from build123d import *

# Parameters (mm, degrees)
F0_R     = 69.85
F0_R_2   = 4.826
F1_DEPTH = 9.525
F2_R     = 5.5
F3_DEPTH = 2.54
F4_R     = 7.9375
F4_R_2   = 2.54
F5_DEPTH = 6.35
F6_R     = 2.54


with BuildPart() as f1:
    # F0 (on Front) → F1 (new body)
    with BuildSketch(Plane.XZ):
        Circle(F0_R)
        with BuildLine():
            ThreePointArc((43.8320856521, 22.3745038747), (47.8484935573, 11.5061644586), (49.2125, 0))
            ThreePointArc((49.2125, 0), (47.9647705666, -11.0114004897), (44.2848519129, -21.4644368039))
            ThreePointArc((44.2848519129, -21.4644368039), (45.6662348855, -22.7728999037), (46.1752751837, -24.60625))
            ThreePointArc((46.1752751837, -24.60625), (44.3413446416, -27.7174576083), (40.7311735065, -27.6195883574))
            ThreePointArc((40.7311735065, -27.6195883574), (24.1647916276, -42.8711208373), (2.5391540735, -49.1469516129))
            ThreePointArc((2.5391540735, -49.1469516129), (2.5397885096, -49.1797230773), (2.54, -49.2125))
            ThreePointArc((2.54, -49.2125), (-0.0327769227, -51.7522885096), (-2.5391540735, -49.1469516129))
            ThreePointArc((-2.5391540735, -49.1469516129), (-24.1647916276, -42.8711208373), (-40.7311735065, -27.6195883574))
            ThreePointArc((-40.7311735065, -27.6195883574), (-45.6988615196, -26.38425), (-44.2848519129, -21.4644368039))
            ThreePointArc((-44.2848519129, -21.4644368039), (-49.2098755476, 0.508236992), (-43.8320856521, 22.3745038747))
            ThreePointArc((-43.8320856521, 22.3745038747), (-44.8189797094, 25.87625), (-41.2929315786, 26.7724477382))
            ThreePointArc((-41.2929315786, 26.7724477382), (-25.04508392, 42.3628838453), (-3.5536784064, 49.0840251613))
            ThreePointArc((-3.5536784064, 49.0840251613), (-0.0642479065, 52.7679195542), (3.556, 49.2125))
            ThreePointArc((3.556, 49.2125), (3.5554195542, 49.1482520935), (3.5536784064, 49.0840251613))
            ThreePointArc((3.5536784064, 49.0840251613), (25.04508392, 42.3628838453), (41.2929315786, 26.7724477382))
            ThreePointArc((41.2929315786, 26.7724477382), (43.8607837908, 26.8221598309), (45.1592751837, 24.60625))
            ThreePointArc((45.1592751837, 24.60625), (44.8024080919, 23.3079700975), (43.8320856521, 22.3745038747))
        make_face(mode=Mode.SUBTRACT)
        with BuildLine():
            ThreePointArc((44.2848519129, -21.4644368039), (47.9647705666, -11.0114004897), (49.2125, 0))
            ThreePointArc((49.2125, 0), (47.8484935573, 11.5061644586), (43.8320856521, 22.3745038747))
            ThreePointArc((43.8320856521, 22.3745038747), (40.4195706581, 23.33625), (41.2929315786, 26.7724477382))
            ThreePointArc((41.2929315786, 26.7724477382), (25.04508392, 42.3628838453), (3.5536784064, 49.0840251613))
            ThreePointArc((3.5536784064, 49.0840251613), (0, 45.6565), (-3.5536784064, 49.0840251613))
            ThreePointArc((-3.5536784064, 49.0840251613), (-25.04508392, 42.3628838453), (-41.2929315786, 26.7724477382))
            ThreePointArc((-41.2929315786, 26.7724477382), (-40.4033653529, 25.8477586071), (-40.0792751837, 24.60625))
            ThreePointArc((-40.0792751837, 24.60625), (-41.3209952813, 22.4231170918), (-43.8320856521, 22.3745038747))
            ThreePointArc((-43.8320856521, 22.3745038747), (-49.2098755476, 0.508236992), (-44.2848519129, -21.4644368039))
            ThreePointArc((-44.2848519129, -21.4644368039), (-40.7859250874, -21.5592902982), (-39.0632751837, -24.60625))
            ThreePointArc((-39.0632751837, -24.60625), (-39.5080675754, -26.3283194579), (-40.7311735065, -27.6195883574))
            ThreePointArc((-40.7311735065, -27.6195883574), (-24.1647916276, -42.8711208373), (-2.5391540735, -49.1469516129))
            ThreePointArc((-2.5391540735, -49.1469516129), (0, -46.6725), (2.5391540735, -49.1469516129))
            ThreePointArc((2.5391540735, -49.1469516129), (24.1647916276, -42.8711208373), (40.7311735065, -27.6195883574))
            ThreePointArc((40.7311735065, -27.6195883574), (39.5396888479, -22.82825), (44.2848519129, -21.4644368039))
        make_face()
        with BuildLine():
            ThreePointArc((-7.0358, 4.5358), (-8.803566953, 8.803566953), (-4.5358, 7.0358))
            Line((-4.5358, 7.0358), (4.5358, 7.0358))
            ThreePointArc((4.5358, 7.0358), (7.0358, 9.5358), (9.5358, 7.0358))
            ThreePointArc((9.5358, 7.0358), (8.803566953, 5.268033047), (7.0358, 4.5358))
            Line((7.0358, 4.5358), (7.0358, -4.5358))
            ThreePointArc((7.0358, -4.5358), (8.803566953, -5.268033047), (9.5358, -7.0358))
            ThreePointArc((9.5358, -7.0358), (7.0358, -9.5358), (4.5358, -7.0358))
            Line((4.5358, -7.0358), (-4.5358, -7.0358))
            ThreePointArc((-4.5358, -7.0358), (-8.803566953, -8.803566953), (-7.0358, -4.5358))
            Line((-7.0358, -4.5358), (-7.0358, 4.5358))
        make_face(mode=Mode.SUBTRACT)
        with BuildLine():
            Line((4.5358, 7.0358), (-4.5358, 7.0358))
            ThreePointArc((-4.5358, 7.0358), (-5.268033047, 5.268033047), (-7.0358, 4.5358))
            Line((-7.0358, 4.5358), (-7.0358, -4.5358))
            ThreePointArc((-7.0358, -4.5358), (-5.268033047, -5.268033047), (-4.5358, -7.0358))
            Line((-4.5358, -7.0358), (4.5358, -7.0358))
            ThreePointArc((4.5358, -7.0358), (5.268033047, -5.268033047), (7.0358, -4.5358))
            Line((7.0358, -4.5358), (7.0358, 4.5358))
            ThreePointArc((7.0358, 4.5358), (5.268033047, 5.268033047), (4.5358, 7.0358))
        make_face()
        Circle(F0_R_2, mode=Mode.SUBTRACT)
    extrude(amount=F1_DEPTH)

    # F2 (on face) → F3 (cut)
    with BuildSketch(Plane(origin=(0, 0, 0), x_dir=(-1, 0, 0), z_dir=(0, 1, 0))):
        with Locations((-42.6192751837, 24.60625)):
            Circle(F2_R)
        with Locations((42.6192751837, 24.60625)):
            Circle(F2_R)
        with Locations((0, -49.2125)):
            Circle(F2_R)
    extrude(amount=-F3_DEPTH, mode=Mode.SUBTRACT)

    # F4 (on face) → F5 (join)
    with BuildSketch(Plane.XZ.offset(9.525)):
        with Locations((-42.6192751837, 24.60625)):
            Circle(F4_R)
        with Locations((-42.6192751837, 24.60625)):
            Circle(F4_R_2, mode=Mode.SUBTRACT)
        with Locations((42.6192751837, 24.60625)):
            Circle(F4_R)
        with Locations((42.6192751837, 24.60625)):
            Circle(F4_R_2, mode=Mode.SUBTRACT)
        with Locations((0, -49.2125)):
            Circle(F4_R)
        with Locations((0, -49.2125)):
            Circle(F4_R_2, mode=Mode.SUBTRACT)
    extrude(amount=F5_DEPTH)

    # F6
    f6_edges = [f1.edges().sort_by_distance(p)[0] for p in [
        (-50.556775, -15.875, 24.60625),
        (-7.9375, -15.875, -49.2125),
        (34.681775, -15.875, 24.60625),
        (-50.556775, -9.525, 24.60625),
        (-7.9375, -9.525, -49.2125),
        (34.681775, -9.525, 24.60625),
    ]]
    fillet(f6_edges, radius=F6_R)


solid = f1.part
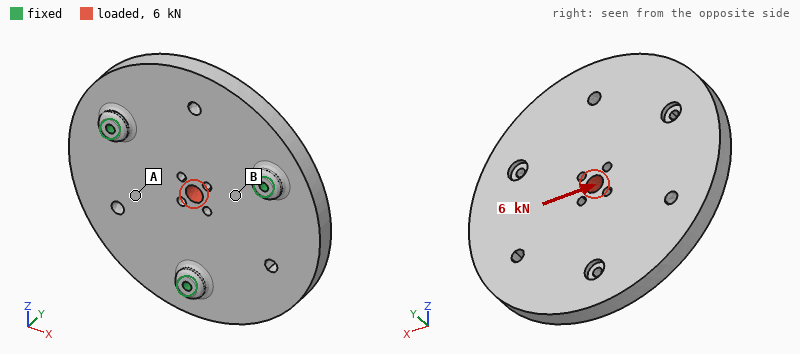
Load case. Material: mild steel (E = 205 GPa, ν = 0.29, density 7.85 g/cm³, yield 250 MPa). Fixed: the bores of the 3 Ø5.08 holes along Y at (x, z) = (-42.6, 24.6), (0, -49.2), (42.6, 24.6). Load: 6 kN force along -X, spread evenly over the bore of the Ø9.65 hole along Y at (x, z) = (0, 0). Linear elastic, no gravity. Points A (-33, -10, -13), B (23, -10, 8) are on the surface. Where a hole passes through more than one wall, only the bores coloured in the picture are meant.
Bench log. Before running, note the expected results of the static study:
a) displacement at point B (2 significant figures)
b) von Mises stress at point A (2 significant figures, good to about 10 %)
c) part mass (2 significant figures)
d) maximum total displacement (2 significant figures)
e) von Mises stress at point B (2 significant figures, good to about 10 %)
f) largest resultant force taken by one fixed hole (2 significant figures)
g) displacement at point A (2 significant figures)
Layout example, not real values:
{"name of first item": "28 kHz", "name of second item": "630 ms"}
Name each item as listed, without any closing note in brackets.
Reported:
{"displacement at point B": "2.5 µm", "von Mises stress at point A": "5.0 MPa", "part mass": "1.1 kg", "maximum total displacement": "5.6 µm", "von Mises stress at point B": "11 MPa", "largest resultant force taken by one fixed hole": "2.2 kN", "displacement at point A": "2.6 µm"}
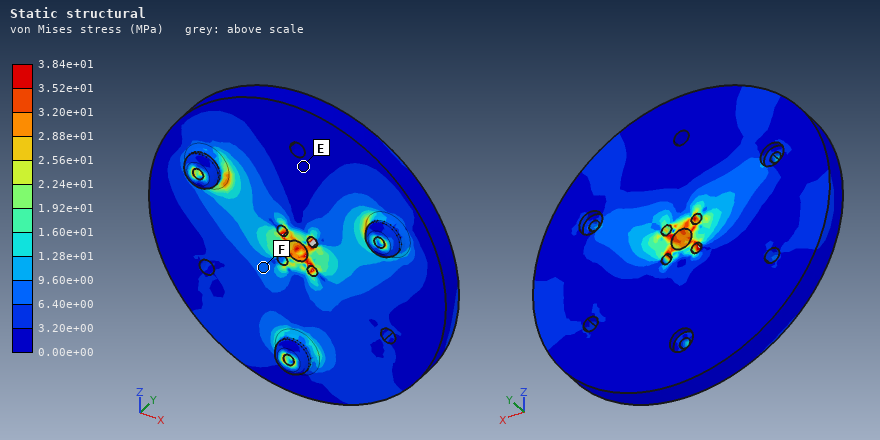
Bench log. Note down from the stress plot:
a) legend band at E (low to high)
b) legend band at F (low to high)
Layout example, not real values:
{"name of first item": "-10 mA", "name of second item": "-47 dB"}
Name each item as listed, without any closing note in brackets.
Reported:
{"legend band at E": "0.00e+00 to 3.20e+00 MPa", "legend band at F": "6.40e+00 to 9.60e+00 MPa"}
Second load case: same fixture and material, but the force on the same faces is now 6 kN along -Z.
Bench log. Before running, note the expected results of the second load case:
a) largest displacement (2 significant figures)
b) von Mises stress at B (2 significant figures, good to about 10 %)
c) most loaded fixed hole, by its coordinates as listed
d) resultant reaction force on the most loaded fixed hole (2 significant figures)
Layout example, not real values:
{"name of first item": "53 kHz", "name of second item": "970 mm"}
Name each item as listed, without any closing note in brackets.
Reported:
{"largest displacement": "6.4 µm", "von Mises stress at B": "6.6 MPa", "most loaded fixed hole, by its coordinates as listed": "(0, -49.2)", "resultant reaction force on the most loaded fixed hole": "2.3 kN"}
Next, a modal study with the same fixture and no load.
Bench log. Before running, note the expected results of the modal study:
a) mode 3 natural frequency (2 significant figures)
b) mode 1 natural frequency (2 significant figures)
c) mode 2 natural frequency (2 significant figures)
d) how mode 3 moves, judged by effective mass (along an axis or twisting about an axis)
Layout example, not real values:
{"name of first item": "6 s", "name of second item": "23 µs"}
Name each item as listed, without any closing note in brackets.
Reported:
{"mode 3 natural frequency": "3900 Hz", "mode 1 natural frequency": "2900 Hz", "mode 2 natural frequency": "2900 Hz", "how mode 3 moves, judged by effective mass": "along Y"}
